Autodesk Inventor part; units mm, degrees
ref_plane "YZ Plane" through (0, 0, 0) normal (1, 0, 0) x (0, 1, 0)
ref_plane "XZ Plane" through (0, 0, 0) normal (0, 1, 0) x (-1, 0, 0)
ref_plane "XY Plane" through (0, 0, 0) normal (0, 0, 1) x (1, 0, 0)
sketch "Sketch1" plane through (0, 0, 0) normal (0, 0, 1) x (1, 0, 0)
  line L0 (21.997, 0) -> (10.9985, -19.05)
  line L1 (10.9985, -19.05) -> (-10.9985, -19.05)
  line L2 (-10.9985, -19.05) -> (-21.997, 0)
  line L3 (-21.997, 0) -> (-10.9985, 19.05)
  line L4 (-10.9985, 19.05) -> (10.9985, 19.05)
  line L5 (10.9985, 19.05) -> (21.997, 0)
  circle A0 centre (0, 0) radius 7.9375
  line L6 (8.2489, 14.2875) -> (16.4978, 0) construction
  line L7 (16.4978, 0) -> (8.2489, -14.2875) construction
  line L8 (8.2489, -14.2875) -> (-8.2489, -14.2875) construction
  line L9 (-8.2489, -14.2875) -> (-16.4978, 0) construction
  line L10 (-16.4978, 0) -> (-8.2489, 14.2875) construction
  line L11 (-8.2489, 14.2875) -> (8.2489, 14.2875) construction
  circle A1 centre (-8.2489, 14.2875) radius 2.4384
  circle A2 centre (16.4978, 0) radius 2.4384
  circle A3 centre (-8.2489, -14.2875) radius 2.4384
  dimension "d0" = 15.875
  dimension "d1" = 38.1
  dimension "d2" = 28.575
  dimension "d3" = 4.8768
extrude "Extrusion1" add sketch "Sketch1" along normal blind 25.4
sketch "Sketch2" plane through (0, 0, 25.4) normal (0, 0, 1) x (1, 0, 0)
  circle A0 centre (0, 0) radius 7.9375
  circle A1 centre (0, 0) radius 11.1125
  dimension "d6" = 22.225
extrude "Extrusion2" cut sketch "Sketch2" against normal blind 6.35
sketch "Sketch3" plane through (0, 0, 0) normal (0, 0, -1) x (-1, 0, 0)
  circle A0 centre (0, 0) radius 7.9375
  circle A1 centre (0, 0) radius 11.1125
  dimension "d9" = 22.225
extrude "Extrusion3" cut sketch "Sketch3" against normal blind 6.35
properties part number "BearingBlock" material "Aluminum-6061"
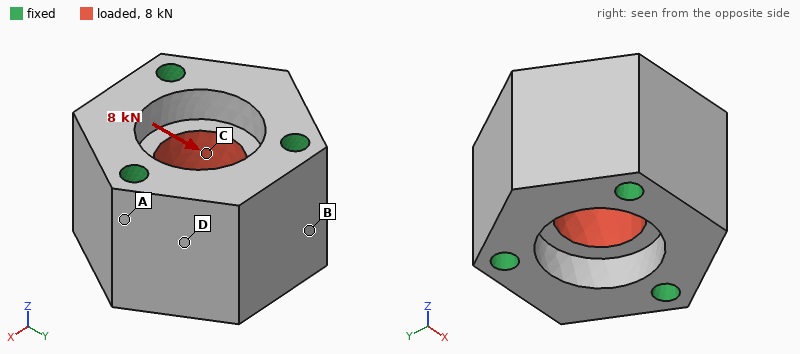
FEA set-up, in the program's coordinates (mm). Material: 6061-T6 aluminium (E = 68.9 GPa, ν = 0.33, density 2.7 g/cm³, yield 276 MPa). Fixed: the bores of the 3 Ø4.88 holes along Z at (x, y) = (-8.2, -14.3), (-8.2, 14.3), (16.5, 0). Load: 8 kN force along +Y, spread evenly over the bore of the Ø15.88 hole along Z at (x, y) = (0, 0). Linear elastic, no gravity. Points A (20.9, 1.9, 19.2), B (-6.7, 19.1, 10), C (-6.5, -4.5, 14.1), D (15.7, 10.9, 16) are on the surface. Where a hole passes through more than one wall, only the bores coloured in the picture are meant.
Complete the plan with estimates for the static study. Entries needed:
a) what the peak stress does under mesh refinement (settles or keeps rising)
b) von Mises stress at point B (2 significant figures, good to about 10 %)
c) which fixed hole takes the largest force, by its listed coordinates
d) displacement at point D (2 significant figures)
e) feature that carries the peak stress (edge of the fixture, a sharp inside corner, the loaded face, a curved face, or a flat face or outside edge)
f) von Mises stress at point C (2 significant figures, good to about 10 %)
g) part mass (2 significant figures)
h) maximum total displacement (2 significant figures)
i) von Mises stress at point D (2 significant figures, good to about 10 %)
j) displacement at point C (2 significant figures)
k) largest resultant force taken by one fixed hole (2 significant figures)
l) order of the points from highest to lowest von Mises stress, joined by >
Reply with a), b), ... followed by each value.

a) keeps rising
b) 6.0 MPa
c) (16.5, 0)
d) 1.4 µm
e) edge of the fixture
f) 20 MPa
g) 62 g
h) 3.4 µm
i) 9.1 MPa
j) 1.8 µm
k) 3.0 kN
l) C > D > B > A
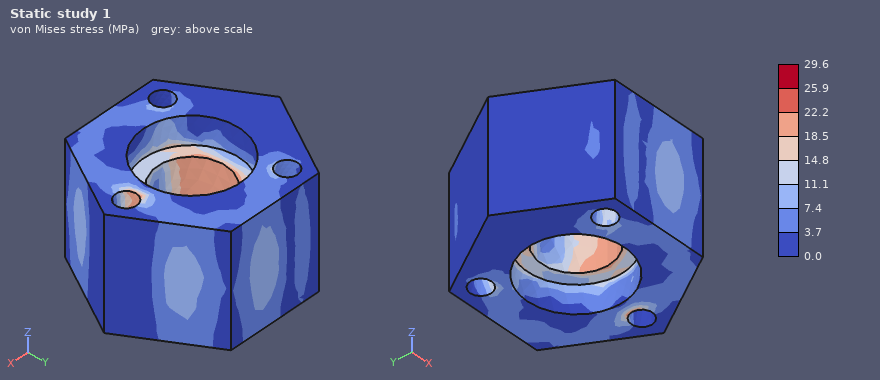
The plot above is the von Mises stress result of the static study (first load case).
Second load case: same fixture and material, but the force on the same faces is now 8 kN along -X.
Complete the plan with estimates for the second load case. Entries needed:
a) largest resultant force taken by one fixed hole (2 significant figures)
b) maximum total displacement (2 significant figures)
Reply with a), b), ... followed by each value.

a) 2.9 kN
b) 3.7 µm
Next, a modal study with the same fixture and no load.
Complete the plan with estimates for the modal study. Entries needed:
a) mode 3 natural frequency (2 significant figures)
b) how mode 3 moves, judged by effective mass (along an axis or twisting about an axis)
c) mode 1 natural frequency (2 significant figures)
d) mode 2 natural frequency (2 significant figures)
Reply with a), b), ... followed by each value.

a) 42 kHz
b) along Z
c) 39 kHz
d) 39 kHz
